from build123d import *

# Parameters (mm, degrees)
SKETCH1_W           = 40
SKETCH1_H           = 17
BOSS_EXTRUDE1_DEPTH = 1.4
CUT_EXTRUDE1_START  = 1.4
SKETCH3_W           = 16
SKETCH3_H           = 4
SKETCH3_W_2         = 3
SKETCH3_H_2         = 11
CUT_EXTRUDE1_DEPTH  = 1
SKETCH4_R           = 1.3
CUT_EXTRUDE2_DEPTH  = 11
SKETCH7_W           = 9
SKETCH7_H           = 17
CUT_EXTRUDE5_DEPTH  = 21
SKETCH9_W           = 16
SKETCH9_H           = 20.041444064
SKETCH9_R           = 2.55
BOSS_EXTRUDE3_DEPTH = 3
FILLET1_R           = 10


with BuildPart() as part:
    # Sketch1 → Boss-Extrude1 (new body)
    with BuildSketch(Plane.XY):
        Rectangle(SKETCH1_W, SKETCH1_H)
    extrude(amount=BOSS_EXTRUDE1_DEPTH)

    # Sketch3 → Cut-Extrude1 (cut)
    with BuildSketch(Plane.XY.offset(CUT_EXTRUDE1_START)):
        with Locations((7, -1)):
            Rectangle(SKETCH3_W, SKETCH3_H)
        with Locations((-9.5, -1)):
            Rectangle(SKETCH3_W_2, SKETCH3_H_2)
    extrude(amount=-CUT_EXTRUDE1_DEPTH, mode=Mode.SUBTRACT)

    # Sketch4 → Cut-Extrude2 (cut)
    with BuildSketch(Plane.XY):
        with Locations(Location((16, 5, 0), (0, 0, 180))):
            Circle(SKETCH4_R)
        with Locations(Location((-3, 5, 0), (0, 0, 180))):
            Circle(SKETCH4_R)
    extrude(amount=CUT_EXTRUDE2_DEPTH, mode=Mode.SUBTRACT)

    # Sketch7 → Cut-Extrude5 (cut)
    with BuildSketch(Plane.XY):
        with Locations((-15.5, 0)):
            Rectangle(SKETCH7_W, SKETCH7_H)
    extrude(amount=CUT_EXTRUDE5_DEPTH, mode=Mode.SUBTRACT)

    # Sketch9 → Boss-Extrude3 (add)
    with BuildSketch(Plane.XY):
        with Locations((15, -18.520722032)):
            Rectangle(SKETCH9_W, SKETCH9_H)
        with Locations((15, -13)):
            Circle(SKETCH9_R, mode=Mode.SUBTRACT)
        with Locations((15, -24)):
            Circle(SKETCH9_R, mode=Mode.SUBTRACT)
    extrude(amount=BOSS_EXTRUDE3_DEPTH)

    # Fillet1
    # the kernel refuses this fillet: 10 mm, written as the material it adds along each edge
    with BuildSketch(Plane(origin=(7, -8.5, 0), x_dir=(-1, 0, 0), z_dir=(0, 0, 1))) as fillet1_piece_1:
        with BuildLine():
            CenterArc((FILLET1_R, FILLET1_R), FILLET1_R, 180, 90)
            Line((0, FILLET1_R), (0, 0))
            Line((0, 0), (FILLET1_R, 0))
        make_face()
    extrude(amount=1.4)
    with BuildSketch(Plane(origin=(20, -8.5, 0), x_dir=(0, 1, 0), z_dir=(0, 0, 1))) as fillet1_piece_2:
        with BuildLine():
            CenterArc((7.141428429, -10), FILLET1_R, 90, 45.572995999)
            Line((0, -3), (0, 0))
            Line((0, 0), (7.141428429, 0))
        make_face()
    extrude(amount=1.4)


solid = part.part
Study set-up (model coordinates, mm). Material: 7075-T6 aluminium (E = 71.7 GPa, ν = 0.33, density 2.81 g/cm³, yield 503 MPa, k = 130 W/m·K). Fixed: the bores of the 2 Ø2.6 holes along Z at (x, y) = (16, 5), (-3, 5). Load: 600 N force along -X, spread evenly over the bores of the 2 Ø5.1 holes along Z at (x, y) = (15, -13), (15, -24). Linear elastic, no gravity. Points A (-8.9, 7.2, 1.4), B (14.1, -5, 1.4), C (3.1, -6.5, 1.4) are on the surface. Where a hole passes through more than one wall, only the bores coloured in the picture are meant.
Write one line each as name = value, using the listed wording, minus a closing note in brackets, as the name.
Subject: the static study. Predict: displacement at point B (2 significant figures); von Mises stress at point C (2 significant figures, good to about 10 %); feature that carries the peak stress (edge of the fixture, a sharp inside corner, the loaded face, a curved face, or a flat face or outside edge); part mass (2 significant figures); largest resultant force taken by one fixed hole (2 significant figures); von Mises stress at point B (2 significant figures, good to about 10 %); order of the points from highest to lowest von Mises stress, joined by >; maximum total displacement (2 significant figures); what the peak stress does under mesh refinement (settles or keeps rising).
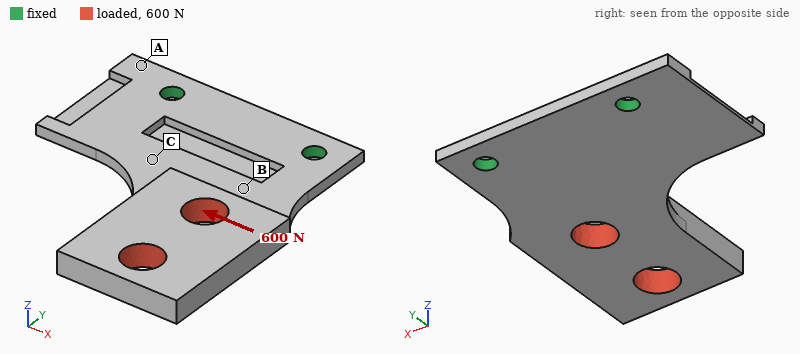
displacement at point B = 0.045 mm
von Mises stress at point C = 110 MPa
feature that carries the peak stress = edge of the fixture
part mass = 4.2 g
largest resultant force taken by one fixed hole = 770 N
von Mises stress at point B = 63 MPa
order of the points from highest to lowest von Mises stress, joined by > = C > B > A
maximum total displacement = 0.26 mm
what the peak stress does under mesh refinement = keeps rising
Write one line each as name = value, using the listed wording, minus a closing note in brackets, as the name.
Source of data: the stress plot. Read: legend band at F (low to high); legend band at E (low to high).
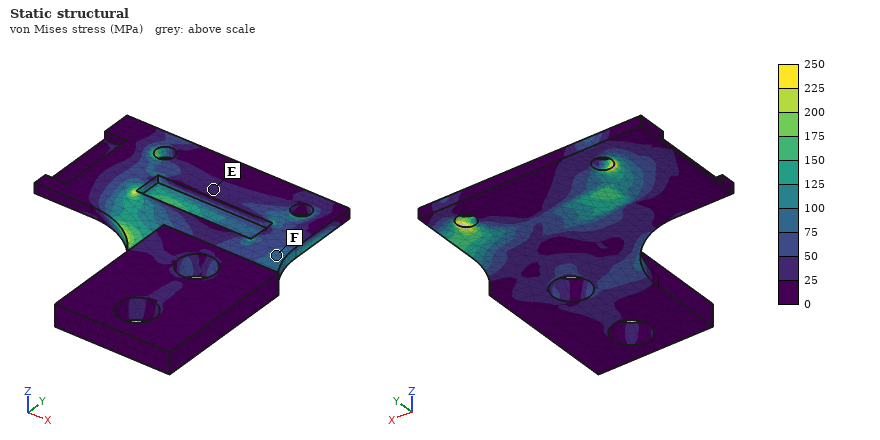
legend band at F = 75 to 100 MPa
legend band at E = 25 to 50 MPa
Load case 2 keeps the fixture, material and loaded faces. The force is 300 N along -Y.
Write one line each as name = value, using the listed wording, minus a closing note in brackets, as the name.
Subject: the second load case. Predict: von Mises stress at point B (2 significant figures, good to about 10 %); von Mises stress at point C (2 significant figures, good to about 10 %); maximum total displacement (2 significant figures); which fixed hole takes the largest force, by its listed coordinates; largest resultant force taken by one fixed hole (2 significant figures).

von Mises stress at point B = 50 MPa
von Mises stress at point C = 43 MPa
maximum total displacement = 0.41 mm
which fixed hole takes the largest force, by its listed coordinates = (16, 5)
largest resultant force taken by one fixed hole = 270 N
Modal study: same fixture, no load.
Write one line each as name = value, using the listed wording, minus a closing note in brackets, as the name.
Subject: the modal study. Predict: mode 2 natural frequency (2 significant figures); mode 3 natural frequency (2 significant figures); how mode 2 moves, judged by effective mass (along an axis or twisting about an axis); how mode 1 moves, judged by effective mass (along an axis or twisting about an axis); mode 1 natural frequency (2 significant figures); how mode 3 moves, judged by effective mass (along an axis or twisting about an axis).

mode 2 natural frequency = 4200 Hz
mode 3 natural frequency = 6800 Hz
how mode 2 moves, judged by effective mass = twisting about Y
how mode 1 moves, judged by effective mass = along Z
mode 1 natural frequency = 770 Hz
how mode 3 moves, judged by effective mass = along Z
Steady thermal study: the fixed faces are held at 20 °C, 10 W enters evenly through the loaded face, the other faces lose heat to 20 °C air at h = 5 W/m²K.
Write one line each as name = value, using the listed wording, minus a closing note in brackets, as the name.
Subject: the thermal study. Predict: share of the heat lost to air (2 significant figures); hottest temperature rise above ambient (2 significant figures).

share of the heat lost to air = 3.3 %
hottest temperature rise above ambient = 69 K
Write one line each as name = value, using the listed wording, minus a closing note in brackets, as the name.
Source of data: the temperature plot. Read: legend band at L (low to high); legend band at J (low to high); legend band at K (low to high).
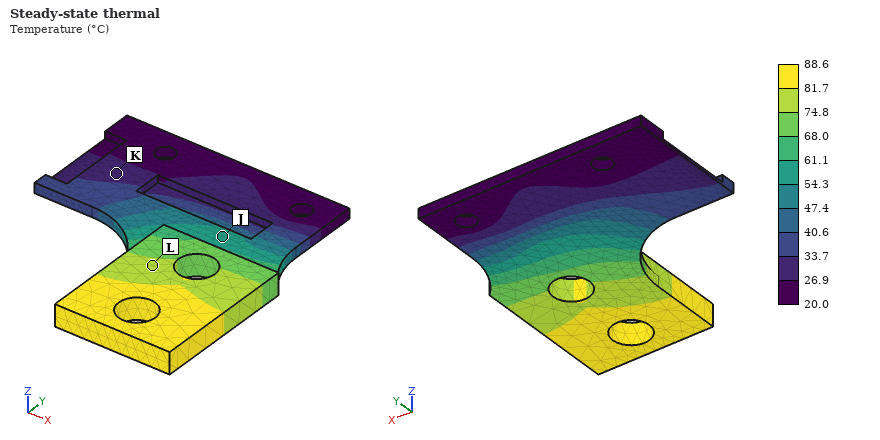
legend band at L = 74.8 to 81.7 °C
legend band at J = 54.3 to 61.1 °C
legend band at K = 26.9 to 33.7 °C
